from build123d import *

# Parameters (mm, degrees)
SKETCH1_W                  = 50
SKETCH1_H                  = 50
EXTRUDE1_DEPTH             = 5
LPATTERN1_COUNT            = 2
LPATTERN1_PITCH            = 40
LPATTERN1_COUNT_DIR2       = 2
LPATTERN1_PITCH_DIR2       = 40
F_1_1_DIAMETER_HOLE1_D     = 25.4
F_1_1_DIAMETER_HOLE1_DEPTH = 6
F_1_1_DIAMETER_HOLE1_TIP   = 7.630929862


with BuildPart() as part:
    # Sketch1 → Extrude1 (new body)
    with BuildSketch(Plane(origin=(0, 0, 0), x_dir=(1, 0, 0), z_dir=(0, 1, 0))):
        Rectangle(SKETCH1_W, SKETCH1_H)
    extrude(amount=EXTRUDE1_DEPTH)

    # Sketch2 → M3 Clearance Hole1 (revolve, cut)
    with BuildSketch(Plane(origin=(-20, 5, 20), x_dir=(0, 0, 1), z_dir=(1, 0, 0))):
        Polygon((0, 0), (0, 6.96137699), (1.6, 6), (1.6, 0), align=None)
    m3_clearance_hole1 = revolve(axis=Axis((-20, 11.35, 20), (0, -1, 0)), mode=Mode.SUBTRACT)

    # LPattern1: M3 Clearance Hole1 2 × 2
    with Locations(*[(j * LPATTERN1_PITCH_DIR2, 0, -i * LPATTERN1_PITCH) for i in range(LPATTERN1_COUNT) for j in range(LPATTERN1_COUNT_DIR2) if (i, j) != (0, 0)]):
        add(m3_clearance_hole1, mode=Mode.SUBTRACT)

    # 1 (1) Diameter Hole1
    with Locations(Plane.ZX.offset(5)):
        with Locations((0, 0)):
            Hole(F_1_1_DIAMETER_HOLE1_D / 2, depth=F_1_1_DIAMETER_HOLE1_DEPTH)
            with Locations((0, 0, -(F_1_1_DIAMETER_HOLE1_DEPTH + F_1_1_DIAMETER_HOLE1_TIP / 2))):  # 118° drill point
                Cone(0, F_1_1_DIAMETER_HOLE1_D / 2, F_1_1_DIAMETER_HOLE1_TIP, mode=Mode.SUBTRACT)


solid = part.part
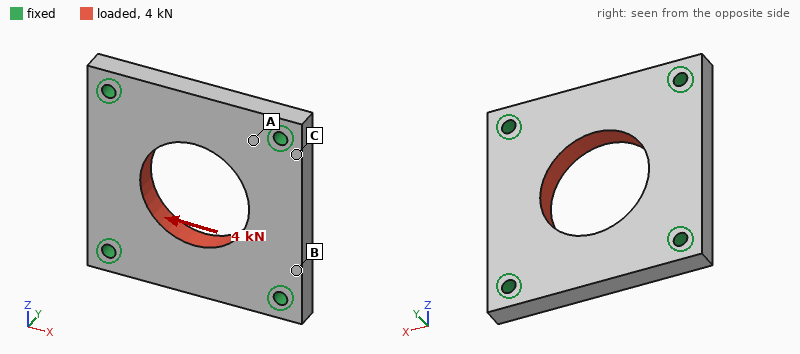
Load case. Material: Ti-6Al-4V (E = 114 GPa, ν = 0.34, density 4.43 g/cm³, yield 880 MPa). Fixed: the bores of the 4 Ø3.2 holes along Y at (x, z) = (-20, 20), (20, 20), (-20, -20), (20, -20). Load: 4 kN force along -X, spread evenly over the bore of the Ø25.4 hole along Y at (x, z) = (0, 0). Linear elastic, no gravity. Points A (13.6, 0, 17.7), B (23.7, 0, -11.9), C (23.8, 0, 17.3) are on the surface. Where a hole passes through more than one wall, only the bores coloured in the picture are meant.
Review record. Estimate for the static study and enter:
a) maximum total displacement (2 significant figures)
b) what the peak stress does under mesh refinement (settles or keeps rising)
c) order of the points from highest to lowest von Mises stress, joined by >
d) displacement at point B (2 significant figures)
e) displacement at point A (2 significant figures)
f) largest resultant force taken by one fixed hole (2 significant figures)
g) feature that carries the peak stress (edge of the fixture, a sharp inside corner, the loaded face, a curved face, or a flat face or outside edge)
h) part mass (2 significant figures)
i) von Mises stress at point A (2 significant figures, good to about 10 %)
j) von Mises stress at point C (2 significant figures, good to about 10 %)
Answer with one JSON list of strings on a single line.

["5.3 µm", "keeps rising", "A > C > B", "2.7 µm", "1.3 µm", "1.1 kN", "edge of the fixture", "43 g", "17 MPa", "11 MPa"]
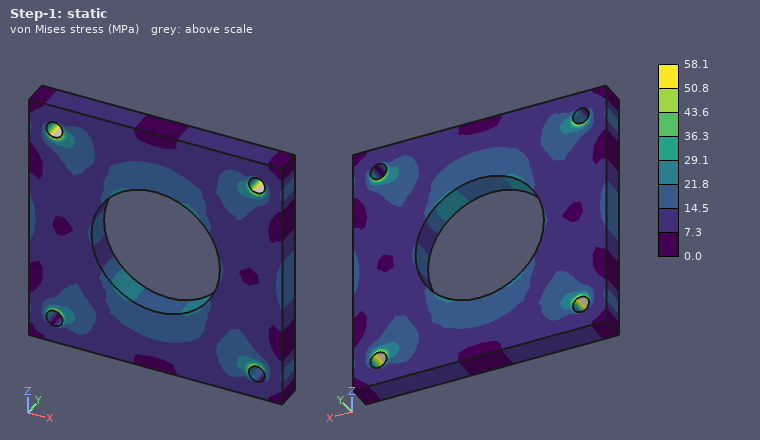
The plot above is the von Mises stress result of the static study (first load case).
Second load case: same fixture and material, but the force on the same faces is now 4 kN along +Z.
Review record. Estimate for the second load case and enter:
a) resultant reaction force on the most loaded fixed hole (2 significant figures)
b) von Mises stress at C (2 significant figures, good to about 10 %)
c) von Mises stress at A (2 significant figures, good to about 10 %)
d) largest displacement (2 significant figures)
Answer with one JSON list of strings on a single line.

["1.1 kN", "8.7 MPa", "15 MPa", "5.3 µm"]
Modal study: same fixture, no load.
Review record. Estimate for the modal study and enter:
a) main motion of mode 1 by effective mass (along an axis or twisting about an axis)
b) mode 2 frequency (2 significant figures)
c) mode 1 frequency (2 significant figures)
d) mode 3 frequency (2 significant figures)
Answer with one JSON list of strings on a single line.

["along Y", "16 kHz", "13 kHz", "16 kHz"]
